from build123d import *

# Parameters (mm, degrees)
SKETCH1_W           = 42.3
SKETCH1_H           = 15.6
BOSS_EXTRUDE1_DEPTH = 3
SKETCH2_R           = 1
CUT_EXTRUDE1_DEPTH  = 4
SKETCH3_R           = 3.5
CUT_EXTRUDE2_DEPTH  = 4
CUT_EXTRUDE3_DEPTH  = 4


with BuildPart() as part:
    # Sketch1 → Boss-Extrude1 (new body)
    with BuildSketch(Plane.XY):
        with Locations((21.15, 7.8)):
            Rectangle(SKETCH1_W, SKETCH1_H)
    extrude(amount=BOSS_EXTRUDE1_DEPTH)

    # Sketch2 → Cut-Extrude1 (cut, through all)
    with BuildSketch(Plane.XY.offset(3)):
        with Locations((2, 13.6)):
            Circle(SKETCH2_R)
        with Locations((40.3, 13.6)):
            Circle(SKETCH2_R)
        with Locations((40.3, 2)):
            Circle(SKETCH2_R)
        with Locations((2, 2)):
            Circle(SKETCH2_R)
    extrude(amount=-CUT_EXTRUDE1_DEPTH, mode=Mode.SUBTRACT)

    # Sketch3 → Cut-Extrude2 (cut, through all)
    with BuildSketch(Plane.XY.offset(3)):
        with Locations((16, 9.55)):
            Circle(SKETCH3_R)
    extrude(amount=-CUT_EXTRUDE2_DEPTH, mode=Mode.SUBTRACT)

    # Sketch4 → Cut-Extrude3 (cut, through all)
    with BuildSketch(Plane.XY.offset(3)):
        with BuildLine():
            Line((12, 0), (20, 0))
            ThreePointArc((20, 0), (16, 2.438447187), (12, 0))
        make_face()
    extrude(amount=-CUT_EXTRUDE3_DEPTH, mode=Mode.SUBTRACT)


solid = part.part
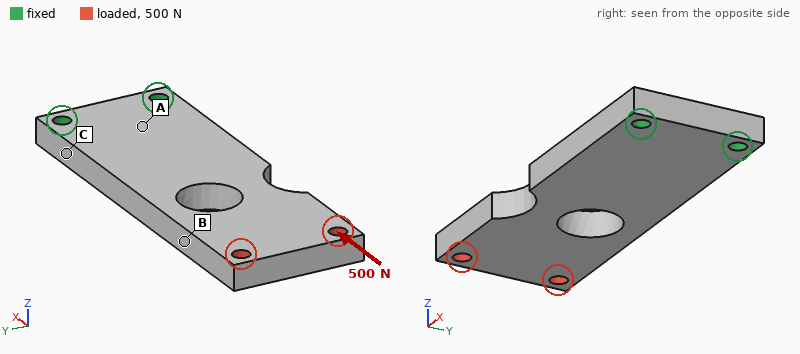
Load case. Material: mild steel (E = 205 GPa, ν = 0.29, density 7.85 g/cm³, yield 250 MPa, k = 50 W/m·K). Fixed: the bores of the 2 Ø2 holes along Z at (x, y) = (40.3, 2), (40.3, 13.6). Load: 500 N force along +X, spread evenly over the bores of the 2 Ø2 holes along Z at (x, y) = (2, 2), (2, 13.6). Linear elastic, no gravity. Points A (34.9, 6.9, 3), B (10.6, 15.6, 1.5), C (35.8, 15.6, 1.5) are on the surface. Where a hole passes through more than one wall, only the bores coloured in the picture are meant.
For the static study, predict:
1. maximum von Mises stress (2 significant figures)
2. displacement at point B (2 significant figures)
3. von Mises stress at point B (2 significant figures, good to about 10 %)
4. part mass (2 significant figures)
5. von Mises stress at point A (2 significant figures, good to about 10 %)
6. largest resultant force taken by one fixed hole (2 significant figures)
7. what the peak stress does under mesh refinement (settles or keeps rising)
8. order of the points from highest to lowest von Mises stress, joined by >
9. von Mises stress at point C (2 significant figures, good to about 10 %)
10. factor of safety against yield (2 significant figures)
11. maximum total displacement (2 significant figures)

51 MPa
2.2 µm
23 MPa
14 g
7.0 MPa
250 N
settles
B > C > A
14 MPa
4.9
3.3 µm
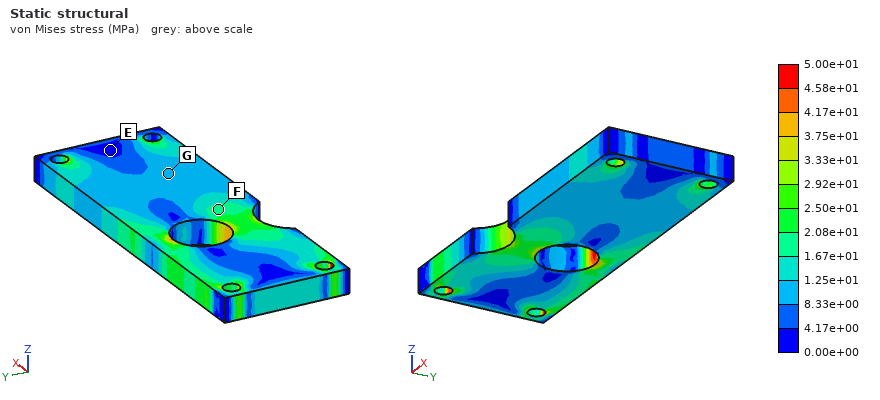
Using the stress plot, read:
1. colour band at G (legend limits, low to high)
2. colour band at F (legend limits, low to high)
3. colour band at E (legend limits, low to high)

8.33e+00 to 1.25e+01 MPa
1.67e+01 to 2.08e+01 MPa
0.00e+00 to 4.17e+00 MPa
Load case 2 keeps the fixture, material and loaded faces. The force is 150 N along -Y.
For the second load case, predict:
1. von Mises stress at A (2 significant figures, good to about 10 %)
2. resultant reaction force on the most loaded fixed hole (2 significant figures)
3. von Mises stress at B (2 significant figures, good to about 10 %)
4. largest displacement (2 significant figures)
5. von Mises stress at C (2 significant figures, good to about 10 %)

8.0 MPa
480 N
15 MPa
21 µm
41 MPa
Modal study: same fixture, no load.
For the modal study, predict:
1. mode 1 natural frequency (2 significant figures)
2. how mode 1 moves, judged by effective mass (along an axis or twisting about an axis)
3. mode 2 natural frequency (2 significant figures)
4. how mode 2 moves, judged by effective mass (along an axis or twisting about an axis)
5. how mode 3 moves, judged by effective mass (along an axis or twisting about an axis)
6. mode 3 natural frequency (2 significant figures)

1500 Hz
along Z
7200 Hz
along Y
twisting about X
7500 Hz
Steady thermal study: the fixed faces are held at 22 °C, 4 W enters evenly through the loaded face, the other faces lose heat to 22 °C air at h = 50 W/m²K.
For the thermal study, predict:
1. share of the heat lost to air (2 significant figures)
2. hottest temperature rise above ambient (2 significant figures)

48 %
58 K
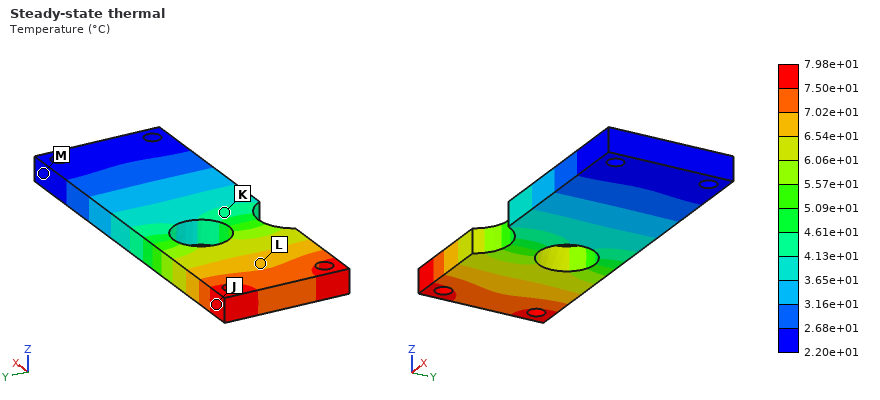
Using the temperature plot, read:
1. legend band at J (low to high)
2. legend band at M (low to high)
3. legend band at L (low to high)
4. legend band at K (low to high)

7.50e+01 to 7.98e+01 °C
2.20e+01 to 2.68e+01 °C
6.54e+01 to 7.02e+01 °C
4.13e+01 to 4.61e+01 °C
